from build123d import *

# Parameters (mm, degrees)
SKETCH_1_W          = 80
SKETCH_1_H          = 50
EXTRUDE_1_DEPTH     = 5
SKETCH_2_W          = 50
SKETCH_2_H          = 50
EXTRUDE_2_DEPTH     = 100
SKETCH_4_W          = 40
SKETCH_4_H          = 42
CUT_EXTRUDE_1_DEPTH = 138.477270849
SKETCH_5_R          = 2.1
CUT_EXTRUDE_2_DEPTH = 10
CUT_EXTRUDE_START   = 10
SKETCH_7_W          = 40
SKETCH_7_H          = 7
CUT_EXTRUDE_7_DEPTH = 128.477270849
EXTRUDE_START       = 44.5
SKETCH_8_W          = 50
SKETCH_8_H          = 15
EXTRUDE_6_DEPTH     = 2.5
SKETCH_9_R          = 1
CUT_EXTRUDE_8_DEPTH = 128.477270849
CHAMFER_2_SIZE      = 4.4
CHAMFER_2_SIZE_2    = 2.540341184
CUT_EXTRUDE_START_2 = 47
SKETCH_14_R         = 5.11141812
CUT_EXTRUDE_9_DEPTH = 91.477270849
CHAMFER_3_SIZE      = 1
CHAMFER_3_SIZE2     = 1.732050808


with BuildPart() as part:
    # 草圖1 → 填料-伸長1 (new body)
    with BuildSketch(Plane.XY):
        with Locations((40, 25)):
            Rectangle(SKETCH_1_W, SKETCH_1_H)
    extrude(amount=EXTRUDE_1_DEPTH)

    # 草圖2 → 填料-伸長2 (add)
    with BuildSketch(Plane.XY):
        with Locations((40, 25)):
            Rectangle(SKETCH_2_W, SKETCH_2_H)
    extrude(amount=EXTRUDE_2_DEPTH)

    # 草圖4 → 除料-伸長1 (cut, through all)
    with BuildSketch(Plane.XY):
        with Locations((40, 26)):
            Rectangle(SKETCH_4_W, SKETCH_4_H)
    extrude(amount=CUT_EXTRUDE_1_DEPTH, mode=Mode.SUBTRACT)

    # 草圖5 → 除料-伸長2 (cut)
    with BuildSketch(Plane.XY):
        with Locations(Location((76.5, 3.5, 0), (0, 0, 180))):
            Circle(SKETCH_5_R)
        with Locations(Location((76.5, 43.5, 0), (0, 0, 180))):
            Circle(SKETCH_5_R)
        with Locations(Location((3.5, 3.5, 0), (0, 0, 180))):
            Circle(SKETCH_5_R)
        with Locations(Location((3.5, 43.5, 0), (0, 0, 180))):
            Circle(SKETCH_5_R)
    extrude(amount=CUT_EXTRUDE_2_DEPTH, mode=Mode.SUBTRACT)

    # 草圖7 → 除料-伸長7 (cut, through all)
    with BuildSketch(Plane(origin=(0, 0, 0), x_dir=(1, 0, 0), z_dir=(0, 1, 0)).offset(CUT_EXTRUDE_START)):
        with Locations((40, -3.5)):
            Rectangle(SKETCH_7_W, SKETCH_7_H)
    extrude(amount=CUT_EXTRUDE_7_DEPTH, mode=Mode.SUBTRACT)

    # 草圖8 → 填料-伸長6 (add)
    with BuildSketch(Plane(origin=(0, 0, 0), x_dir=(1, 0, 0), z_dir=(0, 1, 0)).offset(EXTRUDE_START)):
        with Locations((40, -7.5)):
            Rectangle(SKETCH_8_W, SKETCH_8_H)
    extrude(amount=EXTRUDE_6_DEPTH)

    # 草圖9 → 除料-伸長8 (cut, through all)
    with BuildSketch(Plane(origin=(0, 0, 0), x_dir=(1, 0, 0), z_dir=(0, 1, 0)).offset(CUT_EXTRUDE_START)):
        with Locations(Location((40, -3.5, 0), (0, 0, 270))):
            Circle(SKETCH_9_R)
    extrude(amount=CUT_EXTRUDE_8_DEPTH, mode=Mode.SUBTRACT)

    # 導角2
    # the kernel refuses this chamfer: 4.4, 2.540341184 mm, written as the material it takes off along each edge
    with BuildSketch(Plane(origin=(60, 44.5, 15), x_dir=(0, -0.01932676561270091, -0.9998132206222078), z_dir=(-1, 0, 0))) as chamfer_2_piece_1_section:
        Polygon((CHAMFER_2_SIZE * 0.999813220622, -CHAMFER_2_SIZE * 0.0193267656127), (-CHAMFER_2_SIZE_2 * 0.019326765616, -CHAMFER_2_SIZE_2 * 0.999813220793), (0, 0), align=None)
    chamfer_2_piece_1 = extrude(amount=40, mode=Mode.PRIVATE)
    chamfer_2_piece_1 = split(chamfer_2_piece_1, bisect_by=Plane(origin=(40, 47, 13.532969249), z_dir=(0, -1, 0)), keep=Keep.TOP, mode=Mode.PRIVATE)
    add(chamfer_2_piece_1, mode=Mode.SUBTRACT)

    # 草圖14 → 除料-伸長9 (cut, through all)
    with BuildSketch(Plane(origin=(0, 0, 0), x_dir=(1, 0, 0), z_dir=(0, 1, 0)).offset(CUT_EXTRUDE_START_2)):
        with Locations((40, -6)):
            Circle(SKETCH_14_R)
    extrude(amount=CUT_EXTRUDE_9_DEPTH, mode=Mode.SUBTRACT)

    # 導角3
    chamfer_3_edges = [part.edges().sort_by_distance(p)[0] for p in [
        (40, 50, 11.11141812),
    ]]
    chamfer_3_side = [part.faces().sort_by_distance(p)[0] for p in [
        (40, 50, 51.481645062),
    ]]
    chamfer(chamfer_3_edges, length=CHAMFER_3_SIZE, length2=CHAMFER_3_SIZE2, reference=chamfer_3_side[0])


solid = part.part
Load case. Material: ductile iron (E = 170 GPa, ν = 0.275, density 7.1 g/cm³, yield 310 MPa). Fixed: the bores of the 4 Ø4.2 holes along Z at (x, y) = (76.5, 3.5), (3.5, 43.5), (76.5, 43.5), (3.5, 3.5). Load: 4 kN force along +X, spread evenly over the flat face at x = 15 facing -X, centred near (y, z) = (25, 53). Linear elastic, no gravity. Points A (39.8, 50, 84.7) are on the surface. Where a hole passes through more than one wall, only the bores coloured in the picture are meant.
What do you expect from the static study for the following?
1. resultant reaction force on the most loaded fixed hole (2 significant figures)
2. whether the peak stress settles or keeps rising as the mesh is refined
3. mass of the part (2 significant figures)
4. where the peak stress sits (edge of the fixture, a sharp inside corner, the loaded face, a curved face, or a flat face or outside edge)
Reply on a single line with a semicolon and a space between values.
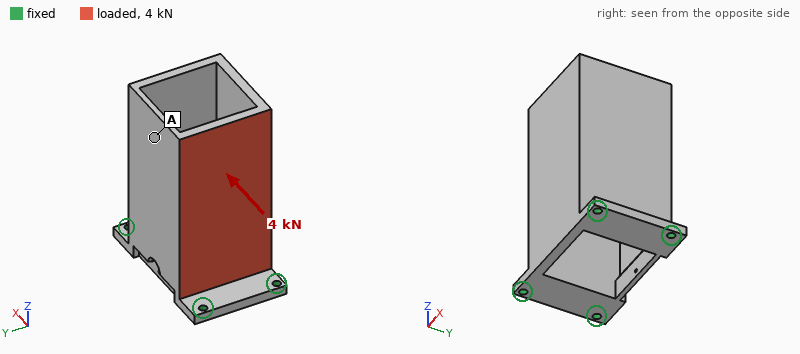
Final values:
2.0 kN; keeps rising; 640 g; edge of the fixture
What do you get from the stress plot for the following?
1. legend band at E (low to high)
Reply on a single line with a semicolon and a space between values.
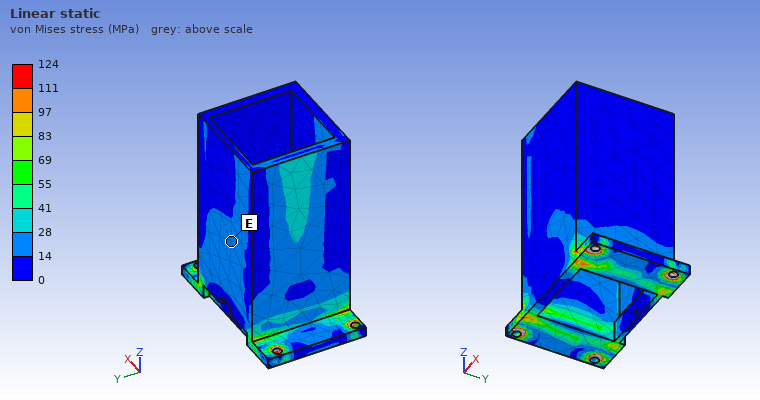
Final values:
14 to 28 MPa
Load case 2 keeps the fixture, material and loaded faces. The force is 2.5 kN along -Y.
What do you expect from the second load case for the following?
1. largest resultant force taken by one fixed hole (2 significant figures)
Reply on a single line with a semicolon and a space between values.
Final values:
2.3 kN
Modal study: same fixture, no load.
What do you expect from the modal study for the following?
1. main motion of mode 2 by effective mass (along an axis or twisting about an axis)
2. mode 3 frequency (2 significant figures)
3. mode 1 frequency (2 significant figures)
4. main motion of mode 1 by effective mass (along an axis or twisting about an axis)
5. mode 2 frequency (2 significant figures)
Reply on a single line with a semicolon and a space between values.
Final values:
along X; 3200 Hz; 1200 Hz; along Y; 1700 Hz
